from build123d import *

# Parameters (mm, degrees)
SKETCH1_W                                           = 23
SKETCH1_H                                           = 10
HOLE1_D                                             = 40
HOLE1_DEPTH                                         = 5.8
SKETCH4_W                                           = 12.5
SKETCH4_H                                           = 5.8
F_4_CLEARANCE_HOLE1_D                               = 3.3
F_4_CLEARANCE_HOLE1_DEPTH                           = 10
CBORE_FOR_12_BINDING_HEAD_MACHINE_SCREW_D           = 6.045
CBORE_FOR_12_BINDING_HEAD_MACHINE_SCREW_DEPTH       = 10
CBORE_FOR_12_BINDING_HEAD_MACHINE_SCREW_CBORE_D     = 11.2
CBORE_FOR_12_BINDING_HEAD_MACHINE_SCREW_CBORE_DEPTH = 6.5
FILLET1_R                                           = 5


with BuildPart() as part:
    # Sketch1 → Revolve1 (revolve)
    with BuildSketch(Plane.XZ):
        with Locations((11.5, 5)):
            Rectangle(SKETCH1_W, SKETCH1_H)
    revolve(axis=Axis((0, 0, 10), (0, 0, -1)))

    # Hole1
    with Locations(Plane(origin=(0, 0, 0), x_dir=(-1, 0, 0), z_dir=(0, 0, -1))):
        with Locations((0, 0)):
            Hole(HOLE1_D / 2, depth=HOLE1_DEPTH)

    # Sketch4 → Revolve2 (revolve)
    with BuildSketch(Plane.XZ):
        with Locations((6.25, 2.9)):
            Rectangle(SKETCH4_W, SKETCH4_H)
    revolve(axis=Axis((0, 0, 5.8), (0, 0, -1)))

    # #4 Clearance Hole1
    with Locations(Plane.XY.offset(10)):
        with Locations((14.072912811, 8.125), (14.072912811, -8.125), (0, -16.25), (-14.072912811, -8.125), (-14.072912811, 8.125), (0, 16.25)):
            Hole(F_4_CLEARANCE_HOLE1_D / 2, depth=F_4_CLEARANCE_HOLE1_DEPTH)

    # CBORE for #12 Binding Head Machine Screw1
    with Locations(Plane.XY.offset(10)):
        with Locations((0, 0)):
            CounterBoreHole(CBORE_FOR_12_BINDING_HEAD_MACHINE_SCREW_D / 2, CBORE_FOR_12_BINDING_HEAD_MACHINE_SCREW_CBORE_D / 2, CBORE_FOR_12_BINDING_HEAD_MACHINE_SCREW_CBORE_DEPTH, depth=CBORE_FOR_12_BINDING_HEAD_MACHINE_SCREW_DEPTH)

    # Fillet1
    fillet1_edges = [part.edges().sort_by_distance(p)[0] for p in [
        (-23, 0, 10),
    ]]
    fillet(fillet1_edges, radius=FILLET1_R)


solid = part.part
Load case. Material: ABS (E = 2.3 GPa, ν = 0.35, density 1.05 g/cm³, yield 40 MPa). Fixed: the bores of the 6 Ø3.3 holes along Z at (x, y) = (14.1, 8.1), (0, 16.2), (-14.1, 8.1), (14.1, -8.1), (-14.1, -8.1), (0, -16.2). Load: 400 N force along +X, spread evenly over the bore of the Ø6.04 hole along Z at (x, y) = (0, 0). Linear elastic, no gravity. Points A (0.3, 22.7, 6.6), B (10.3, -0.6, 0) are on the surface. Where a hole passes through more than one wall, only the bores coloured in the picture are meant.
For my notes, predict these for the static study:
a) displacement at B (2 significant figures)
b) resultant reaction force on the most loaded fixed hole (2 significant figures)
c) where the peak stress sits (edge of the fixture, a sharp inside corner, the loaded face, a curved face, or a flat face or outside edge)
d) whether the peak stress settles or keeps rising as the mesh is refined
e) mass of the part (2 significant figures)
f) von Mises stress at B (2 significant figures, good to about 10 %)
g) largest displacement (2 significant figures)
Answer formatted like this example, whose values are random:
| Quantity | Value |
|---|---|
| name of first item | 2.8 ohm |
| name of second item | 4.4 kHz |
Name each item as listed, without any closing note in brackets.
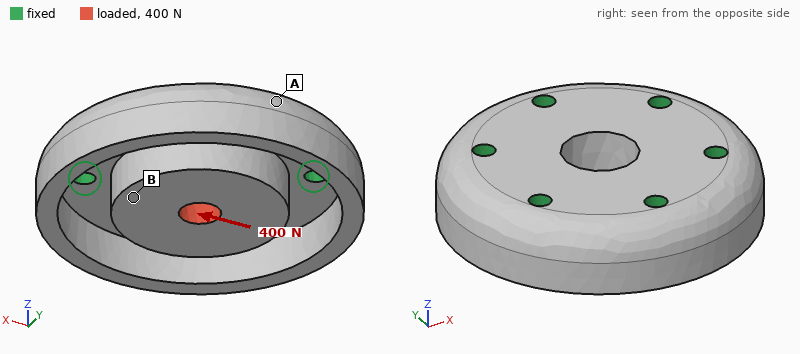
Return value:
| Quantity | Value |
|---|---|
| displacement at B | 23 µm |
| resultant reaction force on the most loaded fixed hole | 96 N |
| where the peak stress sits | a sharp inside corner |
| whether the peak stress settles or keeps rising as the mesh is refined | keeps rising |
| mass of the part | 11 g |
| von Mises stress at B | 2.3 MPa |
| largest displacement | 35 µm |
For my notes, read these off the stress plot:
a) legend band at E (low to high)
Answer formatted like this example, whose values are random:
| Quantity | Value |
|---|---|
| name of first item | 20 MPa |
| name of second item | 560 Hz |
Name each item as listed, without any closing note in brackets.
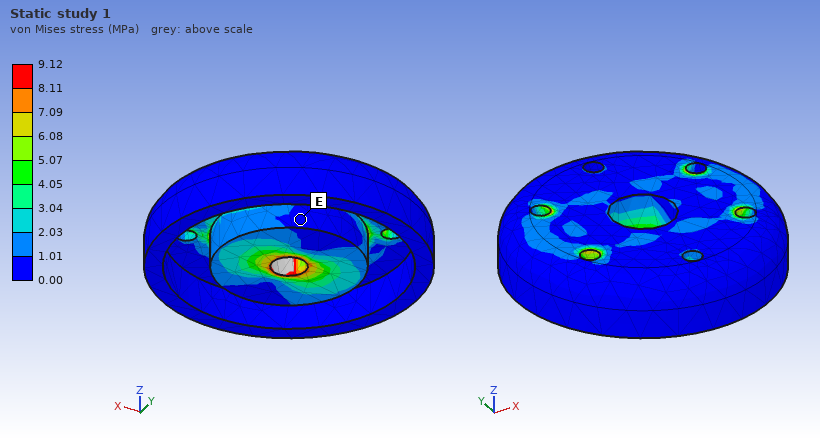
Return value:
| Quantity | Value |
|---|---|
| legend band at E | 0.00 to 1.01 MPa |
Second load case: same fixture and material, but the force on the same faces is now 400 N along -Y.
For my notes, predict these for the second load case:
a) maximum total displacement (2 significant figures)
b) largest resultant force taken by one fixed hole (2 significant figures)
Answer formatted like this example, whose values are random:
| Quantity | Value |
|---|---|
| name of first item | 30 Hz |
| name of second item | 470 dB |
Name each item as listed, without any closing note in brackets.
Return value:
| Quantity | Value |
|---|---|
| maximum total displacement | 35 µm |
| largest resultant force taken by one fixed hole | 110 N |
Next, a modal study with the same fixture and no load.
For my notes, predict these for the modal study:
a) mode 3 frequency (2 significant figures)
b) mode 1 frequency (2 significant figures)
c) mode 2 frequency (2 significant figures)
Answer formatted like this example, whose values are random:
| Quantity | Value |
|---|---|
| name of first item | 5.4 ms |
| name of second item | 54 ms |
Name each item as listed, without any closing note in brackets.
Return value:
| Quantity | Value |
|---|---|
| mode 3 frequency | 8200 Hz |
| mode 1 frequency | 8100 Hz |
| mode 2 frequency | 8100 Hz |
